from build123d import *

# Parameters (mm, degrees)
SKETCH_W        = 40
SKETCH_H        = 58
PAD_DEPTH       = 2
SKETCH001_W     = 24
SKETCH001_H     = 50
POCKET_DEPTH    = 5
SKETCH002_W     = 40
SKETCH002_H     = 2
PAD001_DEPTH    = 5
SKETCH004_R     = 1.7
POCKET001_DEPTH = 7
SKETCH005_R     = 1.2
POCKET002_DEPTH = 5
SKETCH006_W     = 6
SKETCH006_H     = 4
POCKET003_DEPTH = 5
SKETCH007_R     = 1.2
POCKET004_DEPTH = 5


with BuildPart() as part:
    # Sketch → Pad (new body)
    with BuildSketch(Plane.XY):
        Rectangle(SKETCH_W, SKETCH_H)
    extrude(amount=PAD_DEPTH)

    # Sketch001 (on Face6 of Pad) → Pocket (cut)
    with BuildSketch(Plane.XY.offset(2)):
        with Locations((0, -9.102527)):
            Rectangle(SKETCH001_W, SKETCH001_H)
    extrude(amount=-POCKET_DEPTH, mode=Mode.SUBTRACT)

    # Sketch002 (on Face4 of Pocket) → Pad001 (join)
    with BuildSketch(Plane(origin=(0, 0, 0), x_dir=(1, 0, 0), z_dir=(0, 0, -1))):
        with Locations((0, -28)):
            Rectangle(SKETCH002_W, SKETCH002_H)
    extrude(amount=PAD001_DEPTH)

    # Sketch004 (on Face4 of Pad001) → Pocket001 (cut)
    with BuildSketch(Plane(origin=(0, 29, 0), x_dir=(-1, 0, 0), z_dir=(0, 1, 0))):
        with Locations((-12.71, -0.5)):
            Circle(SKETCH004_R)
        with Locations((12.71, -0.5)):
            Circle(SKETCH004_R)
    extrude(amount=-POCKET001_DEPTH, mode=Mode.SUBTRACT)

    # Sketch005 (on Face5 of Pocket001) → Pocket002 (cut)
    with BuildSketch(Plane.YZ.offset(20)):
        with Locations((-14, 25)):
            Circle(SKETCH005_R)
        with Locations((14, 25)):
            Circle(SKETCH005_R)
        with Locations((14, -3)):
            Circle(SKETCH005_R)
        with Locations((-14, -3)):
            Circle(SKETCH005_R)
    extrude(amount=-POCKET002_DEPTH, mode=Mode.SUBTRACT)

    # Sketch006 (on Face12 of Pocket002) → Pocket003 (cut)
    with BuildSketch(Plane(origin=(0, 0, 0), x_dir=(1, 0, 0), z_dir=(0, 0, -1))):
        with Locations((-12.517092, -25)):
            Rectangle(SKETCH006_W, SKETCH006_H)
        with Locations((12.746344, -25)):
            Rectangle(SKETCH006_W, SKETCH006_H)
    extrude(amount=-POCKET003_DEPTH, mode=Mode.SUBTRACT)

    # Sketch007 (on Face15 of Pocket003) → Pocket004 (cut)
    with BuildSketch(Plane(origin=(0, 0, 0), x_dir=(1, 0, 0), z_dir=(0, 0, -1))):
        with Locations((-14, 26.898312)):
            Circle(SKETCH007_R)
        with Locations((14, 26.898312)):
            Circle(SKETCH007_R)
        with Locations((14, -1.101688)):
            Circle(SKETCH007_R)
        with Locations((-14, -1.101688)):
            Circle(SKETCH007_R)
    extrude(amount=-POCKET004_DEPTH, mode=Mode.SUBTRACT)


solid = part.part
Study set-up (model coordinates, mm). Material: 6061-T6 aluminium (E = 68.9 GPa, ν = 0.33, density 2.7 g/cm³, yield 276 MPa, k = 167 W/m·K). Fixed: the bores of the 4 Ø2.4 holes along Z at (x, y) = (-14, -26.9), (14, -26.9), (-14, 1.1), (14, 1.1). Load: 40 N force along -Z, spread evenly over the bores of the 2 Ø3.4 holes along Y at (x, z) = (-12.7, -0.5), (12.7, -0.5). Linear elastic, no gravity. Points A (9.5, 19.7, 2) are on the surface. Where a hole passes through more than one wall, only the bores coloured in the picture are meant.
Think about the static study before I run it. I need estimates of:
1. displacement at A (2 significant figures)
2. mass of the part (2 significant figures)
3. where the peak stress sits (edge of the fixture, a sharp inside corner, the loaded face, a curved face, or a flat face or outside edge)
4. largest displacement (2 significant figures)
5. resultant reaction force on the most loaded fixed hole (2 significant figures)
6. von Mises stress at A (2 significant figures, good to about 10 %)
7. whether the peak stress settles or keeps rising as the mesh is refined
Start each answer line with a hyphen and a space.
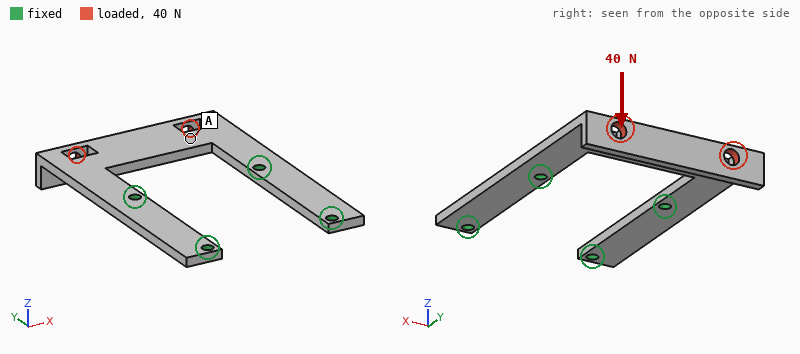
- 0.19 mm
- 7.3 g
- edge of the fixture
- 0.37 mm
- 21 N
- 13 MPa
- keeps rising
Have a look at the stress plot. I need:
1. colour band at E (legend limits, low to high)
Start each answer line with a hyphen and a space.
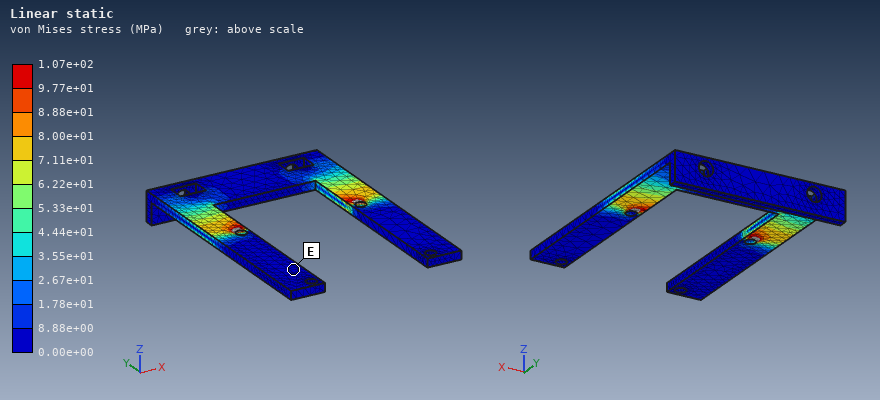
- 0.00e+00 to 8.88e+00 MPa
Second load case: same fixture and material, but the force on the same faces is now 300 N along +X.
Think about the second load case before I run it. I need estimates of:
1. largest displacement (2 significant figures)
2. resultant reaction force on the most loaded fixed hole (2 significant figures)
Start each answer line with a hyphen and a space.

- 97 µm
- 200 N
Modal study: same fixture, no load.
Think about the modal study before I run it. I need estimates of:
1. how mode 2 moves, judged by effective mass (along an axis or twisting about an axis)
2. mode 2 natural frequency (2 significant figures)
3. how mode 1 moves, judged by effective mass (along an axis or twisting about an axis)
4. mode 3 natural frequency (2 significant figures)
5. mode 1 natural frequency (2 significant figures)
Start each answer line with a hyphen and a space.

- twisting about Y
- 2800 Hz
- along Z
- 7400 Hz
- 1100 Hz
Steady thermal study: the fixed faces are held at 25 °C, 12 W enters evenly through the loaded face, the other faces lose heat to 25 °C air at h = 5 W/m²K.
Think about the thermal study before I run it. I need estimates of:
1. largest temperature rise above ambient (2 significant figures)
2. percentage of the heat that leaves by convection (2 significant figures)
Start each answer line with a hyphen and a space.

- 60 K
- 3.7 %
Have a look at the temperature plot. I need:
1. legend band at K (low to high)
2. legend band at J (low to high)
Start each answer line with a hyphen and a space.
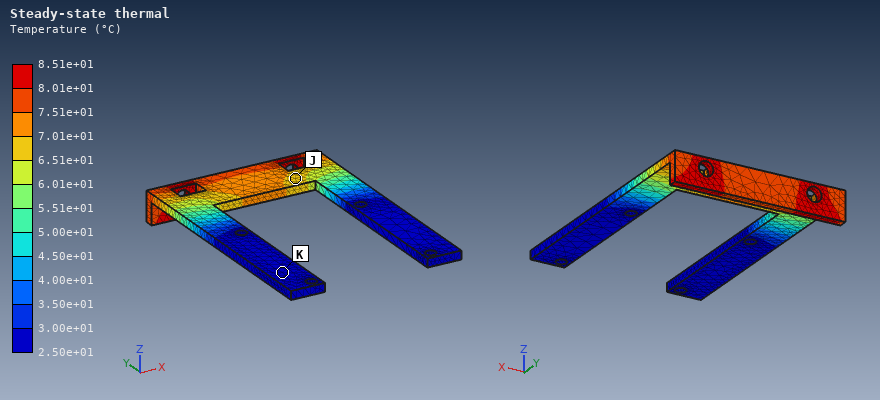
- 2.50e+01 to 3.00e+01 °C
- 6.51e+01 to 7.01e+01 °C
